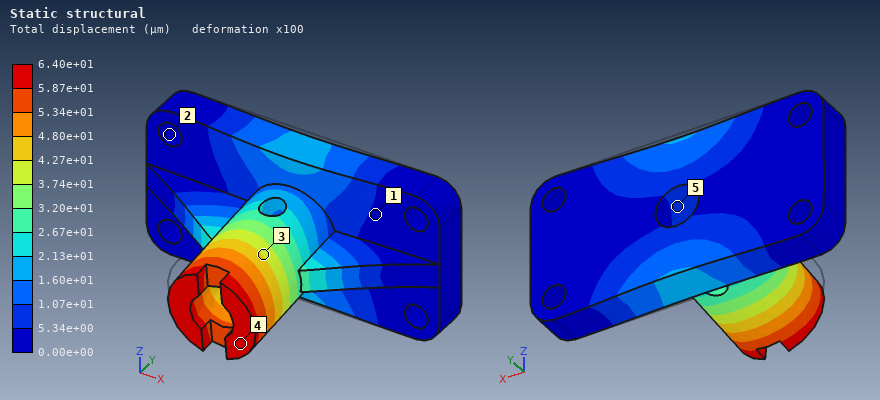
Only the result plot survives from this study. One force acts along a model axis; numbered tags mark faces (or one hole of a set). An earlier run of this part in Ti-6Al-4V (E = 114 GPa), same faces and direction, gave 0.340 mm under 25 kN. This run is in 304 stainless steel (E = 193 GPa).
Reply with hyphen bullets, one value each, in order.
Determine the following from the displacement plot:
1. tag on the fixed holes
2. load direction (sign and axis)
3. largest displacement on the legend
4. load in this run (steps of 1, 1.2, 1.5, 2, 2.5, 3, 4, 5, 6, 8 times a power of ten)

- 2
- -Z
- 6.40e+01 µm
- 8 kN
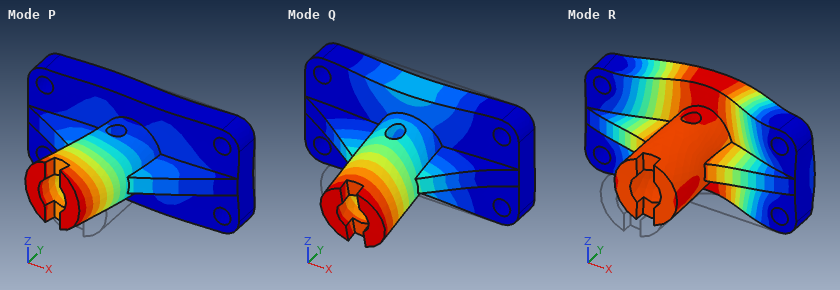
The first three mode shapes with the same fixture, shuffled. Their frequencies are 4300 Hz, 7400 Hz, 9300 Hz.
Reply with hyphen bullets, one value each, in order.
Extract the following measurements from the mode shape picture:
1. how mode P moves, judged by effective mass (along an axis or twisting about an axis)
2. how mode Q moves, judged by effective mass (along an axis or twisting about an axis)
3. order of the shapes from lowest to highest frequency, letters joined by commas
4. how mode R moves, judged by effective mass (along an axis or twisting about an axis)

- along X
- along Z
- Q, R, P
- along Y
